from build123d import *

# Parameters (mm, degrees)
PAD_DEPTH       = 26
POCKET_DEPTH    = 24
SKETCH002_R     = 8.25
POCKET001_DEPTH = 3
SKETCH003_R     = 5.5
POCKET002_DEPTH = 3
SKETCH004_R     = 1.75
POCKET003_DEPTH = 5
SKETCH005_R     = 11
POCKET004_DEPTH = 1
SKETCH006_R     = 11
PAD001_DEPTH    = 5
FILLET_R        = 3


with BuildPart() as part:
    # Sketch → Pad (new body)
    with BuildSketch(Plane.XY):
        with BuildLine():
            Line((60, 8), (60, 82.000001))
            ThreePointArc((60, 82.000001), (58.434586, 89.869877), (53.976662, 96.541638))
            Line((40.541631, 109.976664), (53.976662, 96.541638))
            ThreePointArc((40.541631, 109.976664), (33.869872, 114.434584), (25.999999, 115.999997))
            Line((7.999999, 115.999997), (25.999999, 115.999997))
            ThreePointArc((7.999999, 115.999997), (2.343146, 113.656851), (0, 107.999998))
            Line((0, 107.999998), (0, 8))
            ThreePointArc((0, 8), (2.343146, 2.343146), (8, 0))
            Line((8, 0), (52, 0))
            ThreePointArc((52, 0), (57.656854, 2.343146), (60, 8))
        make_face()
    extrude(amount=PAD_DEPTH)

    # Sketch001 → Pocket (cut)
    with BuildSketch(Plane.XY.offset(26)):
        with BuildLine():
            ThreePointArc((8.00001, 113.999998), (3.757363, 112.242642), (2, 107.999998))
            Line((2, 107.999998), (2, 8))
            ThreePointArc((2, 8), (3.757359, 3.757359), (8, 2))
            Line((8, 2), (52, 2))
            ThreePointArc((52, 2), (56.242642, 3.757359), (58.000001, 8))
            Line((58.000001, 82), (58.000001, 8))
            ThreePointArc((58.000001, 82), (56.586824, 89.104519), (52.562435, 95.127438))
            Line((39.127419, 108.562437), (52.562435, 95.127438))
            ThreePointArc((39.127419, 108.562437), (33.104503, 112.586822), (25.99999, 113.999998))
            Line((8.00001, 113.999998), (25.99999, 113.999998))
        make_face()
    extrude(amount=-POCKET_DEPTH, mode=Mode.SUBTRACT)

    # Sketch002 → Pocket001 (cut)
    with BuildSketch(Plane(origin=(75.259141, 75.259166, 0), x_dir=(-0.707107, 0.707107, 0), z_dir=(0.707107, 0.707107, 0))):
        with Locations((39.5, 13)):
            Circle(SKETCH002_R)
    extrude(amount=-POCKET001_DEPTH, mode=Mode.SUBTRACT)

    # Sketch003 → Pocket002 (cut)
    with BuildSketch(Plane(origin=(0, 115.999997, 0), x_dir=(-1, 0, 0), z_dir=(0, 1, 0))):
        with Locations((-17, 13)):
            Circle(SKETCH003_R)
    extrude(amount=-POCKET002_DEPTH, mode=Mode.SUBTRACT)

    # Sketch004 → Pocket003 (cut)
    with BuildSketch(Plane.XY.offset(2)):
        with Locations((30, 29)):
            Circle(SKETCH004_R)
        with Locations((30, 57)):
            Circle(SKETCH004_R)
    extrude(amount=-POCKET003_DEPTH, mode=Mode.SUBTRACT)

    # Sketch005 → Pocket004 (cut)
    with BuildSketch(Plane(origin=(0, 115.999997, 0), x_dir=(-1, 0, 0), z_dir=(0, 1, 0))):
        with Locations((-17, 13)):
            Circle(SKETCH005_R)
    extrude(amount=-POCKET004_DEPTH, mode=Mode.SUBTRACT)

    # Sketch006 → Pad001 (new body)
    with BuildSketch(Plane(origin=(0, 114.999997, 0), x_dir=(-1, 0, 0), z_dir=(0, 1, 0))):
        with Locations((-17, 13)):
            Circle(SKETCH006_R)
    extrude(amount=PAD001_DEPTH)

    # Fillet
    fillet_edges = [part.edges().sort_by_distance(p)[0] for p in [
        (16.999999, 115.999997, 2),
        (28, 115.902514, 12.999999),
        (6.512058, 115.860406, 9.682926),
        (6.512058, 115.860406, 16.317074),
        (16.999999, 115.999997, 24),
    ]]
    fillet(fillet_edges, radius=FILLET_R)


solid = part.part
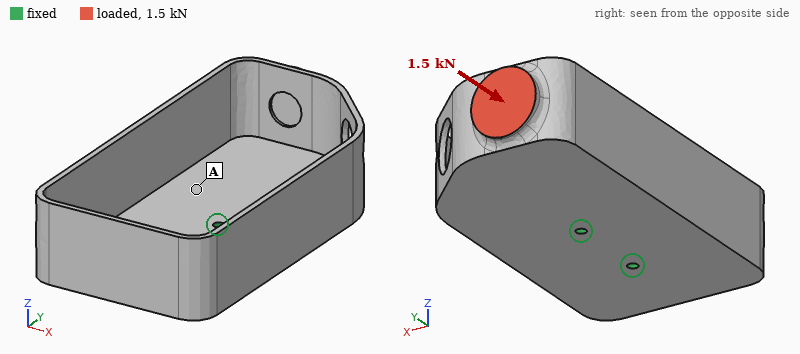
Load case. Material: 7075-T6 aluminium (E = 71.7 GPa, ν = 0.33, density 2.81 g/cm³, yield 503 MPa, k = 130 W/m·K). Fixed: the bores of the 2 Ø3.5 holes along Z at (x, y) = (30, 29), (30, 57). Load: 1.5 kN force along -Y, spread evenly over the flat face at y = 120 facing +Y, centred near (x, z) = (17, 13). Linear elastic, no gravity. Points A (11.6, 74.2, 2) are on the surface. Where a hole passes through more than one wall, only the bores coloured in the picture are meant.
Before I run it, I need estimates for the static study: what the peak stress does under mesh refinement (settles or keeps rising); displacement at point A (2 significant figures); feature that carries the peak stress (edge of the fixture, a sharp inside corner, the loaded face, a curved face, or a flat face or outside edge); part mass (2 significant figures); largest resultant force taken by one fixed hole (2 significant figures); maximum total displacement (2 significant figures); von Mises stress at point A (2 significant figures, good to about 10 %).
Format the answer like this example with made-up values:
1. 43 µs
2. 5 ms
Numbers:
1. keeps rising
2. 0.40 mm
3. edge of the fixture
4. 83 g
5. 1.2 kN
6. 1.3 mm
7. 23 MPa
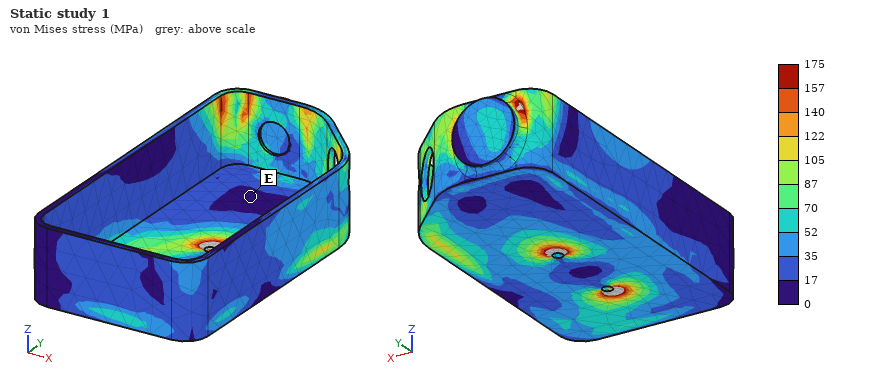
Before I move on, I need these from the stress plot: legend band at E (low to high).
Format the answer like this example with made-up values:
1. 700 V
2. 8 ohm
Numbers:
1. 0 to 17 MPa
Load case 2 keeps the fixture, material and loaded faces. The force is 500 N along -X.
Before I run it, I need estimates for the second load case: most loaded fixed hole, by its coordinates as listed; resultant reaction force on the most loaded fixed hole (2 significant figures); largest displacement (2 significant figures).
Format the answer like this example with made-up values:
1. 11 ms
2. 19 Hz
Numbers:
1. (30, 57)
2. 1.5 kN
3. 0.87 mm
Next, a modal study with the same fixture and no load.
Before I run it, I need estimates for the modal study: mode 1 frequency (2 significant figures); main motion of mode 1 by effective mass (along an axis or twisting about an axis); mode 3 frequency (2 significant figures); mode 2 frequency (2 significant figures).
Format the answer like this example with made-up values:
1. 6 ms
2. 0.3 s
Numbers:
1. 450 Hz
2. along Z
3. 930 Hz
4. 550 Hz
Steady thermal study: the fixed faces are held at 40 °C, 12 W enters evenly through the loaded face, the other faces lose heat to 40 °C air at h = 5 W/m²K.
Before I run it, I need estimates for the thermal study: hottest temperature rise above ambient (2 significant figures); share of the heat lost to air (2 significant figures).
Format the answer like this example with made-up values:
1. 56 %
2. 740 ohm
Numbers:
1. 43 K
2. 17 %
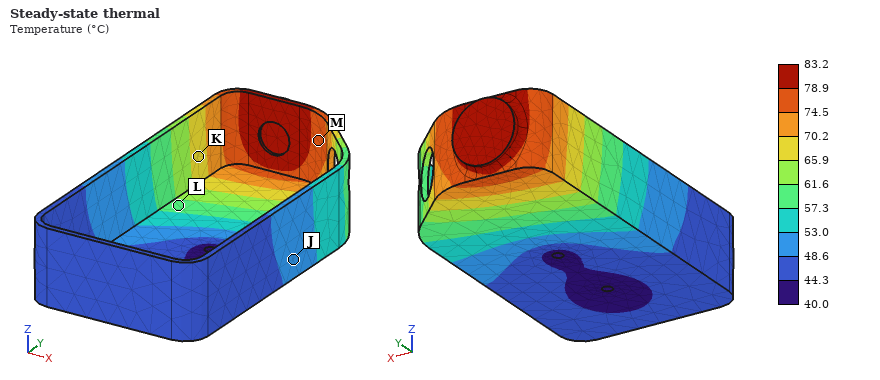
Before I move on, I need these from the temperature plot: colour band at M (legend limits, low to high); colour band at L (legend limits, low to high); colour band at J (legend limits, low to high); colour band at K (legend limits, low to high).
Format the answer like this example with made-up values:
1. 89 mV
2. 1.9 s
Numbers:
1. 74.5 to 78.9 °C
2. 57.3 to 61.6 °C
3. 48.6 to 53.0 °C
4. 65.9 to 70.2 °C
